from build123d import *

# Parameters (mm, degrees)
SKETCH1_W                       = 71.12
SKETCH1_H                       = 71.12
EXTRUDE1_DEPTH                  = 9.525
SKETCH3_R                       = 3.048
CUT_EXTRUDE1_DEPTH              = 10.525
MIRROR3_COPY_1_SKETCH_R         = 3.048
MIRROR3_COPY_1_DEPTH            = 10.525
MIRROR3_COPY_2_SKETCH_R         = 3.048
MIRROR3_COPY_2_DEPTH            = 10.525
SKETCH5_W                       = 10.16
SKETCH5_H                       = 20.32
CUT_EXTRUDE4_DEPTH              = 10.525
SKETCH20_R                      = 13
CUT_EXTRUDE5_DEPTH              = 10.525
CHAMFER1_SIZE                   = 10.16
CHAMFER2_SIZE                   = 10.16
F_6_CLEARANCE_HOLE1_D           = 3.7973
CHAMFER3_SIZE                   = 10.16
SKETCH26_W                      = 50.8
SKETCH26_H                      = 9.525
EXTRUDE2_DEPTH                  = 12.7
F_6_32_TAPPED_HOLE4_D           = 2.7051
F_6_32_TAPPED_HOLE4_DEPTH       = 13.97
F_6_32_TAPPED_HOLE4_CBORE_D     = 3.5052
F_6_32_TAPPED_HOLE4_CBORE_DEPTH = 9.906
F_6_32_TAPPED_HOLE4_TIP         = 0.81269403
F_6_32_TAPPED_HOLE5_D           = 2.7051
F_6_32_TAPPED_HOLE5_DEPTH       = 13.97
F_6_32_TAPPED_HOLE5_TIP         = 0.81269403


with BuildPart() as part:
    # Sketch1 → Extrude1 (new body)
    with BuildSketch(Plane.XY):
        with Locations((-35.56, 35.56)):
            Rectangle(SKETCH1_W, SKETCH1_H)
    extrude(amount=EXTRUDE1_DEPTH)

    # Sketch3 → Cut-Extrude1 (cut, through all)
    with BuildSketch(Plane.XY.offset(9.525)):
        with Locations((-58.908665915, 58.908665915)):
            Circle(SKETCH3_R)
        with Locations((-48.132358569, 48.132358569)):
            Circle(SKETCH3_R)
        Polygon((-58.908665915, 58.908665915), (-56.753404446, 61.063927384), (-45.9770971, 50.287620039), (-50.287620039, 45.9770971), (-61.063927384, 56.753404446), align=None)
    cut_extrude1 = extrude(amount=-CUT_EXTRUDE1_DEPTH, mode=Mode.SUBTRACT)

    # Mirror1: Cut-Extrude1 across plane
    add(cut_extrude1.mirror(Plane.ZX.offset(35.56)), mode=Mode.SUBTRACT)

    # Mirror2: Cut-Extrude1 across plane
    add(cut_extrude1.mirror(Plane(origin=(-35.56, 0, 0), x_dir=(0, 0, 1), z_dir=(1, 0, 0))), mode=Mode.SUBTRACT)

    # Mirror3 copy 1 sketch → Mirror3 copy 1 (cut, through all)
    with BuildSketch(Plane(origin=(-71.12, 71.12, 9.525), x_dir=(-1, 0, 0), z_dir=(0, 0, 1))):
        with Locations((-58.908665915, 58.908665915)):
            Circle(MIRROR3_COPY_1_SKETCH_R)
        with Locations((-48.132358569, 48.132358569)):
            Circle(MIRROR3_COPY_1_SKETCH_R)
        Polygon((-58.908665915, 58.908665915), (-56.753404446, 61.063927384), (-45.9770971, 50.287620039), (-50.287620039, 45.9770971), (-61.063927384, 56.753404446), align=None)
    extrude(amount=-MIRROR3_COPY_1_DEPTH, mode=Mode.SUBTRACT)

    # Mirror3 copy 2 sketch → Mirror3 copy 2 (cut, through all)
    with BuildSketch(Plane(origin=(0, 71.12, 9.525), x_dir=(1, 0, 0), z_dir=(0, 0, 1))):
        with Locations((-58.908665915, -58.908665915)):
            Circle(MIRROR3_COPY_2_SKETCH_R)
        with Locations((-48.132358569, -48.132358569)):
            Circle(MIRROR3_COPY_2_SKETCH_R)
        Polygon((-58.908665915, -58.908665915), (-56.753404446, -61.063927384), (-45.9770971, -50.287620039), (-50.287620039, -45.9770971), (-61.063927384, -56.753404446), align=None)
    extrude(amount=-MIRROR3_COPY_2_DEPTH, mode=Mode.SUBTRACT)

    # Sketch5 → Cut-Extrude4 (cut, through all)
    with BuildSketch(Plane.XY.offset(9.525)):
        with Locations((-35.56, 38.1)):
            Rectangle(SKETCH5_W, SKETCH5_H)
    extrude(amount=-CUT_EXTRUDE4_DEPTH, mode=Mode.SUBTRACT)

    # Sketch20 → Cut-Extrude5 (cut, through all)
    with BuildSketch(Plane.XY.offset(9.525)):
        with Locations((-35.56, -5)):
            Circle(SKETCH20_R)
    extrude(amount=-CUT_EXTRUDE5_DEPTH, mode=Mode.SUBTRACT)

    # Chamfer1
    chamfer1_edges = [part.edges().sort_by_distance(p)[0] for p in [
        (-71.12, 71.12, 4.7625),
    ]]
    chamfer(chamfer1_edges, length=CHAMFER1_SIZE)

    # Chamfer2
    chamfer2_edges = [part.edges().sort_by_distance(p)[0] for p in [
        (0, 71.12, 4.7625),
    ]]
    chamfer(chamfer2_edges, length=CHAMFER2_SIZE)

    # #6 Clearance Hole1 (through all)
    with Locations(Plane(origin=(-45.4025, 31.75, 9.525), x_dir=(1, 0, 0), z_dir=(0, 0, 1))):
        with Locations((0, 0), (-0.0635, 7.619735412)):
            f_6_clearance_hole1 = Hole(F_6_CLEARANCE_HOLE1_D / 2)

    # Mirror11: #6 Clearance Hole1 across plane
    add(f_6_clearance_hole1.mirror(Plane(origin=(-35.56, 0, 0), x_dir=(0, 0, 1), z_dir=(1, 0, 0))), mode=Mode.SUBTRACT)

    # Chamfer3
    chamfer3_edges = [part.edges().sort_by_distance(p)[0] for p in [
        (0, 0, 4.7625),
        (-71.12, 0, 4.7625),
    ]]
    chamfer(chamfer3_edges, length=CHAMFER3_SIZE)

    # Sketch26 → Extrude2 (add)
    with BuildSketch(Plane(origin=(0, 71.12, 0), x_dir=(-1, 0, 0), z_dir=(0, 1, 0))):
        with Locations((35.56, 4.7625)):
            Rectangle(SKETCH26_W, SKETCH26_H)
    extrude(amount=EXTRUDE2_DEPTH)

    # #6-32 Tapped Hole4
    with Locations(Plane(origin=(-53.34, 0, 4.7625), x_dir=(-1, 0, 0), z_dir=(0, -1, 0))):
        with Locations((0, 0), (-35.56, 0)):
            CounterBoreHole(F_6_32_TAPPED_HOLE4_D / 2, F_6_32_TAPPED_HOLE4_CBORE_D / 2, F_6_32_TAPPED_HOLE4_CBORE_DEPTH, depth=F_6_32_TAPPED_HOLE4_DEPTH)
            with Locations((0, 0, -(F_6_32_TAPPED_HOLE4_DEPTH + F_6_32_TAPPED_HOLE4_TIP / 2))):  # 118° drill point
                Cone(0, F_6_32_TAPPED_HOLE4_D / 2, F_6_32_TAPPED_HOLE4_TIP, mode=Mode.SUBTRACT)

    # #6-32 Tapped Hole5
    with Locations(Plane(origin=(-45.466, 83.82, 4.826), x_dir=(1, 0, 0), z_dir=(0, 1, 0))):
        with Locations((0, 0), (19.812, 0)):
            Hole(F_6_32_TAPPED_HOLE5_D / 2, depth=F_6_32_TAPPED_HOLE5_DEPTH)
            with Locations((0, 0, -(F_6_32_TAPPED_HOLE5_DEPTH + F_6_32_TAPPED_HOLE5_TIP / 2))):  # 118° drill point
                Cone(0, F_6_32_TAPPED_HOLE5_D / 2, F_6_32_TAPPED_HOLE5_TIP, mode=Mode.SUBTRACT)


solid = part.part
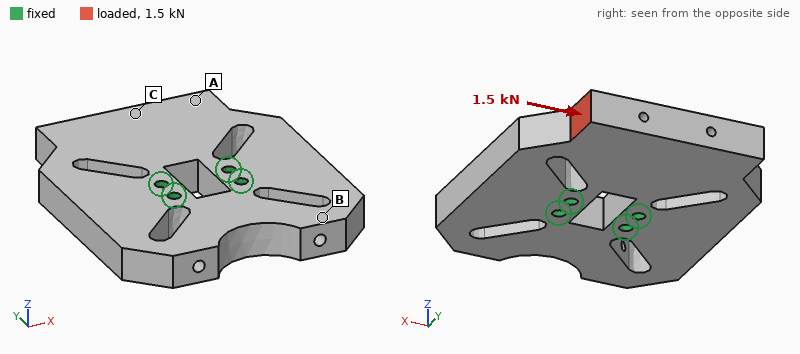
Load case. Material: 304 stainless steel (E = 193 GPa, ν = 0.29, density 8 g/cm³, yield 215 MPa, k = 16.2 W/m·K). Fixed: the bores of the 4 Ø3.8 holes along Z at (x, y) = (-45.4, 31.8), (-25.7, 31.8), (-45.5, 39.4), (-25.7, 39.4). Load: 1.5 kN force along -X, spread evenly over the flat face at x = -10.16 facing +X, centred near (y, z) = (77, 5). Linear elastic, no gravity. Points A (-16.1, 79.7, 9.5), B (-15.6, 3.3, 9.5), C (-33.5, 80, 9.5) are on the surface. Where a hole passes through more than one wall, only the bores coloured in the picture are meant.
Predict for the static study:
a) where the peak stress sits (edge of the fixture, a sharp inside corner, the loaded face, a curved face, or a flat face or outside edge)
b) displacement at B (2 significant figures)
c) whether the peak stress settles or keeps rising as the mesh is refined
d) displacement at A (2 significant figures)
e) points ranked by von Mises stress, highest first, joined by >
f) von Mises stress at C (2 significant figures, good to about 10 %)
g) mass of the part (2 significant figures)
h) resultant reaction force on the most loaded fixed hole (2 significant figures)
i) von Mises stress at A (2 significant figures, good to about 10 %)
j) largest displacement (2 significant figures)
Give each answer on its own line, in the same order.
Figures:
edge of the fixture
2.9 µm
keeps rising
8.5 µm
A > C > B
6.4 MPa
350 g
1.9 kN
12 MPa
9.9 µm
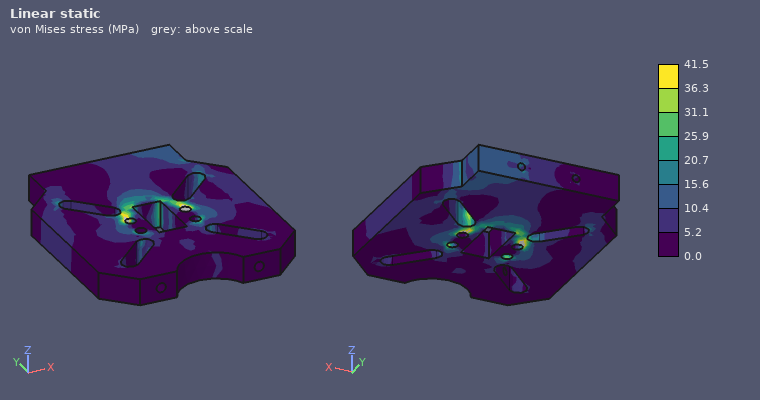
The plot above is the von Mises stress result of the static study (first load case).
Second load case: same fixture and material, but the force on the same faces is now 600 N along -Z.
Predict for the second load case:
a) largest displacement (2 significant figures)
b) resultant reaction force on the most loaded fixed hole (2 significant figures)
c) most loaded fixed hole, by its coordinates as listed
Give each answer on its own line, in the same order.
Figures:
47 µm
1.1 kN
(-25.7, 39.4)
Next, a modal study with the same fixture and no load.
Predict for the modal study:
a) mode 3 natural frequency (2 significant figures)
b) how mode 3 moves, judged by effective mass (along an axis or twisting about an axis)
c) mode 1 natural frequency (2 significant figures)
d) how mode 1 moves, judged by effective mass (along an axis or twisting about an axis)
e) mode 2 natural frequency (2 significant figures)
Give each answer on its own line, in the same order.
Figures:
5700 Hz
along Z
2800 Hz
along Z
5500 Hz
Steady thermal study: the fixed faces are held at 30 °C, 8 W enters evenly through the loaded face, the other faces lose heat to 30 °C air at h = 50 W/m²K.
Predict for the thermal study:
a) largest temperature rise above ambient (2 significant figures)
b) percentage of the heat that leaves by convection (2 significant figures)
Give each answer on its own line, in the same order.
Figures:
67 K
67 %
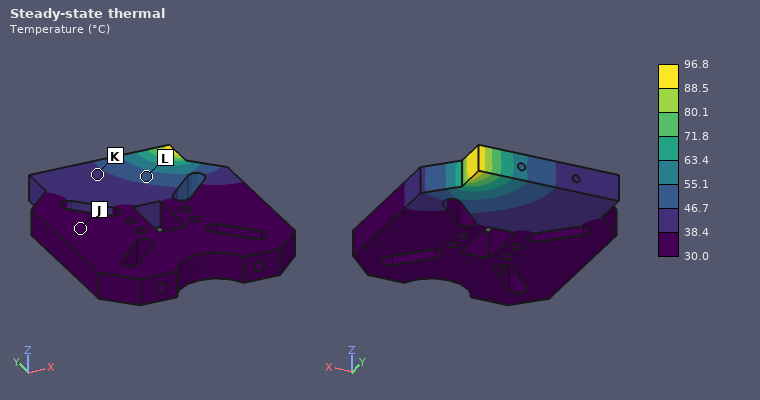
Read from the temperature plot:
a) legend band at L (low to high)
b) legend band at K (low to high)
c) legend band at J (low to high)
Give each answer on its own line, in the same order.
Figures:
46.7 to 55.1 °C
38.4 to 46.7 °C
30.0 to 38.4 °C
